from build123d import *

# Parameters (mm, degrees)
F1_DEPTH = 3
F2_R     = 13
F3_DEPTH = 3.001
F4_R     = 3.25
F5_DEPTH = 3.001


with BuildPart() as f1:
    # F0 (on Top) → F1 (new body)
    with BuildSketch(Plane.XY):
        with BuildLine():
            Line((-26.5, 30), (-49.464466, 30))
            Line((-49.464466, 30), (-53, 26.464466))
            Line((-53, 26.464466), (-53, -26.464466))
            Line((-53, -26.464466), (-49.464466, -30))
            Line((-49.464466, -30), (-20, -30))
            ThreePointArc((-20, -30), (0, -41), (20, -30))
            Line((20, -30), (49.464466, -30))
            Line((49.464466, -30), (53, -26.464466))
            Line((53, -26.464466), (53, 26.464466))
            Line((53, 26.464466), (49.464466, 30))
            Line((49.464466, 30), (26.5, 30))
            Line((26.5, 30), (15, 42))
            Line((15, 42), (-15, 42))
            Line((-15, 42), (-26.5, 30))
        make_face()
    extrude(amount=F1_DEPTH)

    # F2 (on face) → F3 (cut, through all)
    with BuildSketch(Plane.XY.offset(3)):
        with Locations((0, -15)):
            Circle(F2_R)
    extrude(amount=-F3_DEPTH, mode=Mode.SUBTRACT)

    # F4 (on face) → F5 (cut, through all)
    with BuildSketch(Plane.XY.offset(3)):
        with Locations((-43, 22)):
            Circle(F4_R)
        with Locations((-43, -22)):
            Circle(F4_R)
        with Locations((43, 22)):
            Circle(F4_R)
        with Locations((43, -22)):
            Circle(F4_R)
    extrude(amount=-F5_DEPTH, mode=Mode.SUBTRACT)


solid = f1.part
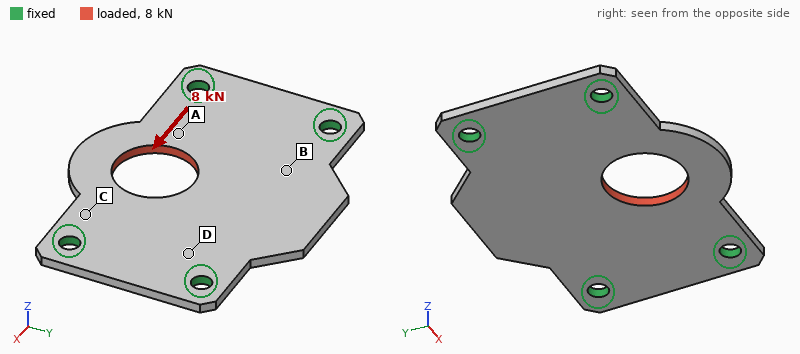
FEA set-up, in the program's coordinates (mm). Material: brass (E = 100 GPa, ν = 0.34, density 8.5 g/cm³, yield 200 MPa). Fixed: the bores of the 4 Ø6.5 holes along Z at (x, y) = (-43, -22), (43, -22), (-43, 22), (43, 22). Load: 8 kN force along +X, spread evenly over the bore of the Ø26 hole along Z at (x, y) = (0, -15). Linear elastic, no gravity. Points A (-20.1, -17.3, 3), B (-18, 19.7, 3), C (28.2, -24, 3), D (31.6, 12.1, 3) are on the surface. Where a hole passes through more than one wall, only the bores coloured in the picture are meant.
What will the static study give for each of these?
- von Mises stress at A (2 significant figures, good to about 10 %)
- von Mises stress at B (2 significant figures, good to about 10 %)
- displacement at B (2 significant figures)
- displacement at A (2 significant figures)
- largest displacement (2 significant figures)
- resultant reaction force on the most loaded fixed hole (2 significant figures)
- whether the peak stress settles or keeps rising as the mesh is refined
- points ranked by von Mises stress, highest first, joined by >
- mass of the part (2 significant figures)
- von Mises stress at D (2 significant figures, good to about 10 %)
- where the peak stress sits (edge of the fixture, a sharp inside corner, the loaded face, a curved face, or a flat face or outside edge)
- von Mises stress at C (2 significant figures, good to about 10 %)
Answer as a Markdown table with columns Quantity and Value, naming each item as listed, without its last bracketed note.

| Quantity | Value |
|---|---|
| von Mises stress at A | 36 MPa |
| von Mises stress at B | 9.5 MPa |
| displacement at B | 3.8 µm |
| displacement at A | 9.9 µm |
| largest displacement | 21 µm |
| resultant reaction force on the most loaded fixed hole | 2.7 kN |
| whether the peak stress settles or keeps rising as the mesh is refined | keeps rising |
| points ranked by von Mises stress, highest first, joined by > | C > A > D > B |
| mass of the part | 170 g |
| von Mises stress at D | 22 MPa |
| where the peak stress sits | edge of the fixture |
| von Mises stress at C | 50 MPa |
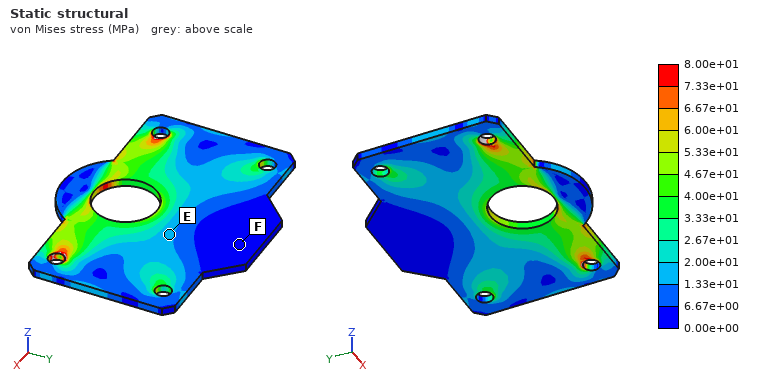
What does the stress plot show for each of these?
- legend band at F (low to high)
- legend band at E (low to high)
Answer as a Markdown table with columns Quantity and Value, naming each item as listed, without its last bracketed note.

| Quantity | Value |
|---|---|
| legend band at F | 0.00e+00 to 6.67e+00 MPa |
| legend band at E | 1.33e+01 to 2.00e+01 MPa |
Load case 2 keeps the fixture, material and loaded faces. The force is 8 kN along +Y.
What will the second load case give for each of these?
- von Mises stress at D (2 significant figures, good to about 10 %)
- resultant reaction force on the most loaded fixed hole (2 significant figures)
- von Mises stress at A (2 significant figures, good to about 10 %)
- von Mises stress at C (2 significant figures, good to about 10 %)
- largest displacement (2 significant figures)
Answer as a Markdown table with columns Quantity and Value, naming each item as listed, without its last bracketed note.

| Quantity | Value |
|---|---|
| von Mises stress at D | 49 MPa |
| resultant reaction force on the most loaded fixed hole | 2.5 kN |
| von Mises stress at A | 53 MPa |
| von Mises stress at C | 29 MPa |
| largest displacement | 39 µm |
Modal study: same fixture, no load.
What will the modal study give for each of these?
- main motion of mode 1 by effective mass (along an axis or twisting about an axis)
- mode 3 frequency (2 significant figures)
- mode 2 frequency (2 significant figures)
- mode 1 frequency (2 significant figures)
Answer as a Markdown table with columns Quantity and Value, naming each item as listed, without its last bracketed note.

| Quantity | Value |
|---|---|
| main motion of mode 1 by effective mass | along Z |
| mode 3 frequency | 2400 Hz |
| mode 2 frequency | 1600 Hz |
| mode 1 frequency | 1300 Hz |
